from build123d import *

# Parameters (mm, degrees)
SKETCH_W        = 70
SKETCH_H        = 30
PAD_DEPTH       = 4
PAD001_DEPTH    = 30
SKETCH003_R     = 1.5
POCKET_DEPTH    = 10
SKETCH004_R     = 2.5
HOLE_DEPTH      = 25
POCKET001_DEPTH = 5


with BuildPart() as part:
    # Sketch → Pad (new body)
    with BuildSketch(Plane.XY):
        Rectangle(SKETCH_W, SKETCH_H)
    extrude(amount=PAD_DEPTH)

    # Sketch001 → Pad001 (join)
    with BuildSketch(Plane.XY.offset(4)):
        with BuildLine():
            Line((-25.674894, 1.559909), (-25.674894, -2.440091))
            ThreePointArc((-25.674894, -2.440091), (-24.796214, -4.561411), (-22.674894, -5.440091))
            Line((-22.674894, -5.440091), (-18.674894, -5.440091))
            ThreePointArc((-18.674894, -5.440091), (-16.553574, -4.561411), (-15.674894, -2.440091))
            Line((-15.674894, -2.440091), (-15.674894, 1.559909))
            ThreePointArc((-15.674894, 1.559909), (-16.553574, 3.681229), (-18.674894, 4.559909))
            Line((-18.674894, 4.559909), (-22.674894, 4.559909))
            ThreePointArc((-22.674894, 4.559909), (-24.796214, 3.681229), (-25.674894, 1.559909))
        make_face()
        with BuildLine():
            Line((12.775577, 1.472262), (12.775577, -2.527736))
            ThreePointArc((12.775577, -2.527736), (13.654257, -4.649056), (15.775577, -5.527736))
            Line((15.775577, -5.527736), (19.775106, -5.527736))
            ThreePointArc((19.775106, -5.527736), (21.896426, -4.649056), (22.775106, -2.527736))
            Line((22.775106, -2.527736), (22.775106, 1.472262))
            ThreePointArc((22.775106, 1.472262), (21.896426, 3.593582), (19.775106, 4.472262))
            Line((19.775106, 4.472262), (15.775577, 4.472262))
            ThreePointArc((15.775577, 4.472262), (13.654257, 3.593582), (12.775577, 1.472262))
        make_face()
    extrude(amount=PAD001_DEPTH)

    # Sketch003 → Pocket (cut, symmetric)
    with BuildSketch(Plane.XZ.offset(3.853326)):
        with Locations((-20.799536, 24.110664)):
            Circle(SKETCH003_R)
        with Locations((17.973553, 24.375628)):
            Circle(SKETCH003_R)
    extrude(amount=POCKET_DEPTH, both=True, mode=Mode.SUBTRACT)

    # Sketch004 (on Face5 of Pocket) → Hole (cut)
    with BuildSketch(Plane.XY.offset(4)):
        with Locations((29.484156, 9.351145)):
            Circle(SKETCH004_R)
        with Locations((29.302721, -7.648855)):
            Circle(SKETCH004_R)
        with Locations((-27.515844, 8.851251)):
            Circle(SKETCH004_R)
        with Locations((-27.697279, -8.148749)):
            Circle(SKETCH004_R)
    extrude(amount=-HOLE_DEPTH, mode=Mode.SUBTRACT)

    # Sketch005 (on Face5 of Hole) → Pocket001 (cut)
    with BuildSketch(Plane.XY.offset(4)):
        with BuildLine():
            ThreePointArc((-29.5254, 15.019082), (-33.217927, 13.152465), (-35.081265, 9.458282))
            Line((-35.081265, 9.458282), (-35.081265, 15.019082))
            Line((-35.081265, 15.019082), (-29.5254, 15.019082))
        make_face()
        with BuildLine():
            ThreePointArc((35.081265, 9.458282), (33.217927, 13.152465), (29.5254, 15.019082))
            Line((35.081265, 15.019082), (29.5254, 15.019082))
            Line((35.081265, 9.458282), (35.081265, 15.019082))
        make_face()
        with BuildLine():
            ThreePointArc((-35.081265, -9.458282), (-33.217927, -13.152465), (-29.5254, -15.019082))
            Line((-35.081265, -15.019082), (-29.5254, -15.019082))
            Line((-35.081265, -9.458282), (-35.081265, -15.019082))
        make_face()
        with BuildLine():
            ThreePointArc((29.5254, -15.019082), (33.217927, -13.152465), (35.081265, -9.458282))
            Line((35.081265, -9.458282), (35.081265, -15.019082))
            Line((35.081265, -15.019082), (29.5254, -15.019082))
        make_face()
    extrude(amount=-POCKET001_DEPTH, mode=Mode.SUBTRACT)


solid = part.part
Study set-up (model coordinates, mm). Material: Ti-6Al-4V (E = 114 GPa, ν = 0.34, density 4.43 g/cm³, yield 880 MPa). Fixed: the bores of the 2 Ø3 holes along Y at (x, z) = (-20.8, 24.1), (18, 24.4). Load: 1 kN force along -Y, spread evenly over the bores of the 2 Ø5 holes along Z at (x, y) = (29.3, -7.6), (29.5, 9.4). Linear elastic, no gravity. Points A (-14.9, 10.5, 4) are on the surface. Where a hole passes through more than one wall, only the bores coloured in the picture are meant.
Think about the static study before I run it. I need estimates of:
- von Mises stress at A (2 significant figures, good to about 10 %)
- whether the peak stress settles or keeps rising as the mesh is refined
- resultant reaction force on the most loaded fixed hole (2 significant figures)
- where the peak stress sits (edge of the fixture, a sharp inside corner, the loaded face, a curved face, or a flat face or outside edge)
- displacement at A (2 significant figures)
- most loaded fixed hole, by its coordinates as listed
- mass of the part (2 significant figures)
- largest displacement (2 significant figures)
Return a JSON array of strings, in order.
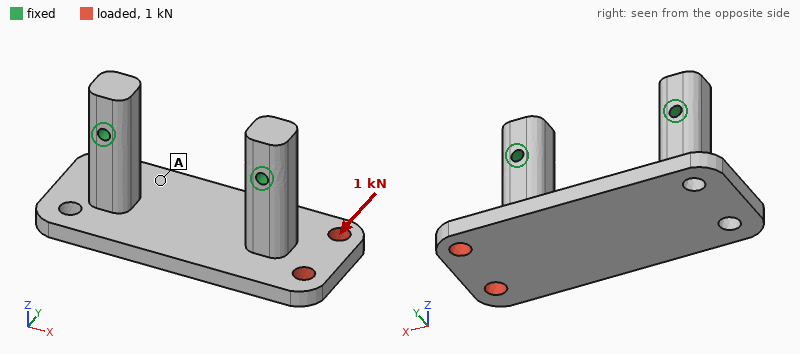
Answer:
["21 MPa", "keeps rising", "1.1 kN", "edge of the fixture", "18 µm", "(18, 24.4)", "59 g", "97 µm"]
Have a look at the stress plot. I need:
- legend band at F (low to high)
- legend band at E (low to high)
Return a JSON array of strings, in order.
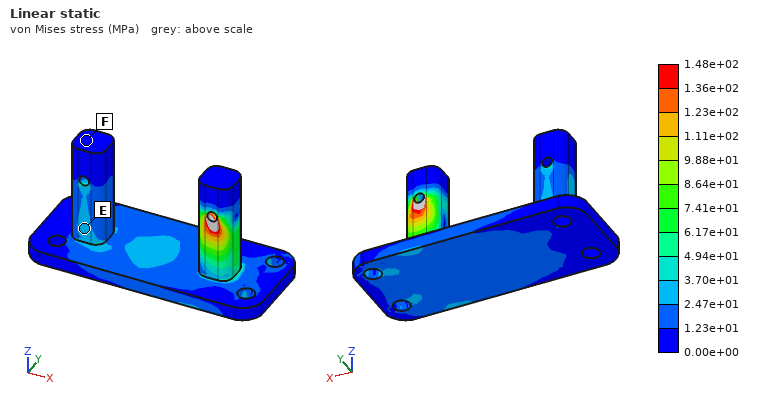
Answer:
["0.00e+00 to 1.23e+01 MPa", "2.47e+01 to 3.70e+01 MPa"]
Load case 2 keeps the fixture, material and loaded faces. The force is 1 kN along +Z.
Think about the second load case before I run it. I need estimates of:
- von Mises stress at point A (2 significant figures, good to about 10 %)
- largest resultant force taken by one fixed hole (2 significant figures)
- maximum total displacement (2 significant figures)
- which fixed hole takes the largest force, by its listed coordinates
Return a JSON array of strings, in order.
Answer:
["13 MPa", "1.2 kN", "75 µm", "(18, 24.4)"]
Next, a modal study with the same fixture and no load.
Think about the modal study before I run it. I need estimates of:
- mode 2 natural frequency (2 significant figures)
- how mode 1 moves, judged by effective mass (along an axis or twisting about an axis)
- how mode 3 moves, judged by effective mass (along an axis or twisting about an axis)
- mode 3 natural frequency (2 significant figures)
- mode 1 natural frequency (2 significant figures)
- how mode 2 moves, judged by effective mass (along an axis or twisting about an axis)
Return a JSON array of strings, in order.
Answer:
["5000 Hz", "along Y", "twisting about Z", "5500 Hz", "4400 Hz", "along X"]
